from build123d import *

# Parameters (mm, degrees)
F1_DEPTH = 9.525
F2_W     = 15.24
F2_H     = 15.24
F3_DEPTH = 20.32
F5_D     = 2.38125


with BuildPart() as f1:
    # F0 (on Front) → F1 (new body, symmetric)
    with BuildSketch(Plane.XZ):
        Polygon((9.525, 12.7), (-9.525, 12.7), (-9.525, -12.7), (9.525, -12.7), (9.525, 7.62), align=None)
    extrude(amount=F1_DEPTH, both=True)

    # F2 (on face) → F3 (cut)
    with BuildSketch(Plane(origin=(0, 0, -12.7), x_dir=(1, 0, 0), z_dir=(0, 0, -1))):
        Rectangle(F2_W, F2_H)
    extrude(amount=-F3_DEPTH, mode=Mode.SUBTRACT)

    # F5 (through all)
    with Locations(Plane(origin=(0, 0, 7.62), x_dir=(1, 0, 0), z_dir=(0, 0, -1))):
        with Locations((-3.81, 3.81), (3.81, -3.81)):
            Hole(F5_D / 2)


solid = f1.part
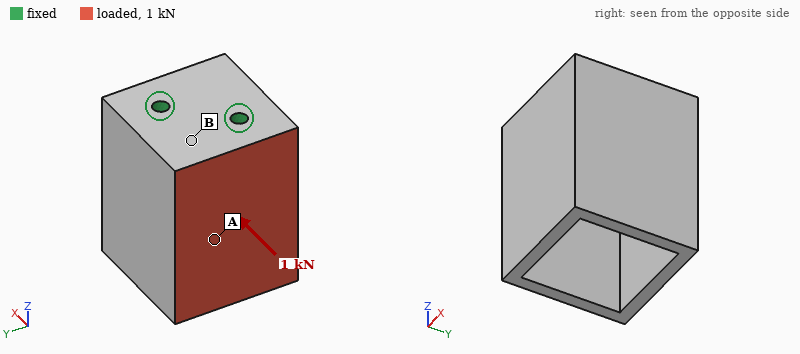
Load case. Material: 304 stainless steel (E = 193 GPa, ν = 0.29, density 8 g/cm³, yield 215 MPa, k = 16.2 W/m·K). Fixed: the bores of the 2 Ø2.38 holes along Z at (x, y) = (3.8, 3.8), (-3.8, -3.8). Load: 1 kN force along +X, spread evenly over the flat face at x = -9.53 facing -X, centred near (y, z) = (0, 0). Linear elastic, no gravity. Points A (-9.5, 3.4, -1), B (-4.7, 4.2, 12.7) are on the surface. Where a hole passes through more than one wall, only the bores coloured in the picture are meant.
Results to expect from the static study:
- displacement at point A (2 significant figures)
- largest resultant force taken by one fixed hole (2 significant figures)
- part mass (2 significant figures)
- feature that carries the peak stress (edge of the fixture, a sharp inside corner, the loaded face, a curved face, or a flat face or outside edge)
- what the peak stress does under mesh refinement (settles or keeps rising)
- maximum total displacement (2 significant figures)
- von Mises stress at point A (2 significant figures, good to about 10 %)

12 µm
690 N
36 g
edge of the fixture
keeps rising
23 µm
32 MPa
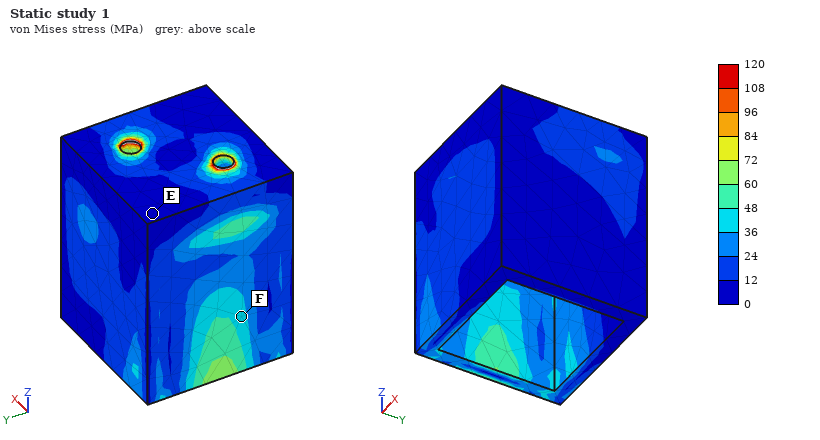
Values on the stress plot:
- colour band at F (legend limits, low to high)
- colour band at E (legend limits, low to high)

36 to 48 MPa
0 to 12 MPa
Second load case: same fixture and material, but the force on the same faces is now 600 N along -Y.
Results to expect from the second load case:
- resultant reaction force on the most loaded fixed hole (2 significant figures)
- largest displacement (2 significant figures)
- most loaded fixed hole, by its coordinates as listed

770 N
13 µm
(-3.8, -3.8)
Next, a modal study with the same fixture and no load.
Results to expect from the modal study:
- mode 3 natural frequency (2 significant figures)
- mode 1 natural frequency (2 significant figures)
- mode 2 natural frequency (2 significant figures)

13 kHz
8200 Hz
12 kHz
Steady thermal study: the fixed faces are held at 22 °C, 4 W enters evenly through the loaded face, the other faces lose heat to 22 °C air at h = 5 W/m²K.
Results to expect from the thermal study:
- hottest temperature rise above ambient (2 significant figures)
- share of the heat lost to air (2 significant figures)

37 K
6.0 %
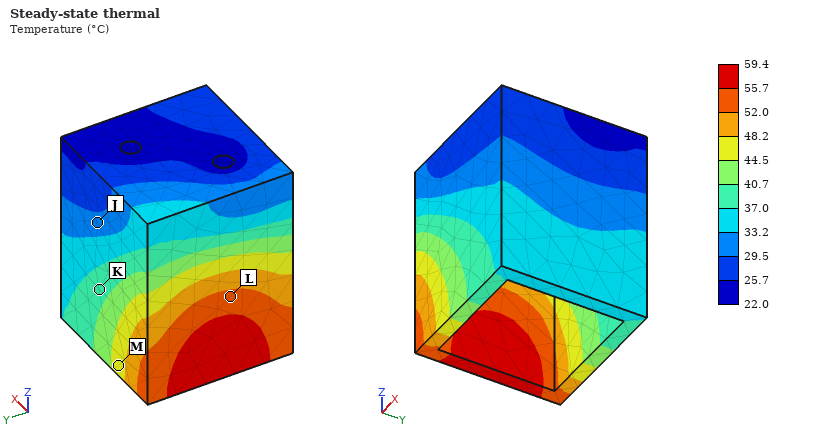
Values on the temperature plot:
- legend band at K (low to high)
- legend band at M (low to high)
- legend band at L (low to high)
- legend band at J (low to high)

37.0 to 40.7 °C
44.5 to 48.2 °C
52.0 to 55.7 °C
29.5 to 33.2 °C
